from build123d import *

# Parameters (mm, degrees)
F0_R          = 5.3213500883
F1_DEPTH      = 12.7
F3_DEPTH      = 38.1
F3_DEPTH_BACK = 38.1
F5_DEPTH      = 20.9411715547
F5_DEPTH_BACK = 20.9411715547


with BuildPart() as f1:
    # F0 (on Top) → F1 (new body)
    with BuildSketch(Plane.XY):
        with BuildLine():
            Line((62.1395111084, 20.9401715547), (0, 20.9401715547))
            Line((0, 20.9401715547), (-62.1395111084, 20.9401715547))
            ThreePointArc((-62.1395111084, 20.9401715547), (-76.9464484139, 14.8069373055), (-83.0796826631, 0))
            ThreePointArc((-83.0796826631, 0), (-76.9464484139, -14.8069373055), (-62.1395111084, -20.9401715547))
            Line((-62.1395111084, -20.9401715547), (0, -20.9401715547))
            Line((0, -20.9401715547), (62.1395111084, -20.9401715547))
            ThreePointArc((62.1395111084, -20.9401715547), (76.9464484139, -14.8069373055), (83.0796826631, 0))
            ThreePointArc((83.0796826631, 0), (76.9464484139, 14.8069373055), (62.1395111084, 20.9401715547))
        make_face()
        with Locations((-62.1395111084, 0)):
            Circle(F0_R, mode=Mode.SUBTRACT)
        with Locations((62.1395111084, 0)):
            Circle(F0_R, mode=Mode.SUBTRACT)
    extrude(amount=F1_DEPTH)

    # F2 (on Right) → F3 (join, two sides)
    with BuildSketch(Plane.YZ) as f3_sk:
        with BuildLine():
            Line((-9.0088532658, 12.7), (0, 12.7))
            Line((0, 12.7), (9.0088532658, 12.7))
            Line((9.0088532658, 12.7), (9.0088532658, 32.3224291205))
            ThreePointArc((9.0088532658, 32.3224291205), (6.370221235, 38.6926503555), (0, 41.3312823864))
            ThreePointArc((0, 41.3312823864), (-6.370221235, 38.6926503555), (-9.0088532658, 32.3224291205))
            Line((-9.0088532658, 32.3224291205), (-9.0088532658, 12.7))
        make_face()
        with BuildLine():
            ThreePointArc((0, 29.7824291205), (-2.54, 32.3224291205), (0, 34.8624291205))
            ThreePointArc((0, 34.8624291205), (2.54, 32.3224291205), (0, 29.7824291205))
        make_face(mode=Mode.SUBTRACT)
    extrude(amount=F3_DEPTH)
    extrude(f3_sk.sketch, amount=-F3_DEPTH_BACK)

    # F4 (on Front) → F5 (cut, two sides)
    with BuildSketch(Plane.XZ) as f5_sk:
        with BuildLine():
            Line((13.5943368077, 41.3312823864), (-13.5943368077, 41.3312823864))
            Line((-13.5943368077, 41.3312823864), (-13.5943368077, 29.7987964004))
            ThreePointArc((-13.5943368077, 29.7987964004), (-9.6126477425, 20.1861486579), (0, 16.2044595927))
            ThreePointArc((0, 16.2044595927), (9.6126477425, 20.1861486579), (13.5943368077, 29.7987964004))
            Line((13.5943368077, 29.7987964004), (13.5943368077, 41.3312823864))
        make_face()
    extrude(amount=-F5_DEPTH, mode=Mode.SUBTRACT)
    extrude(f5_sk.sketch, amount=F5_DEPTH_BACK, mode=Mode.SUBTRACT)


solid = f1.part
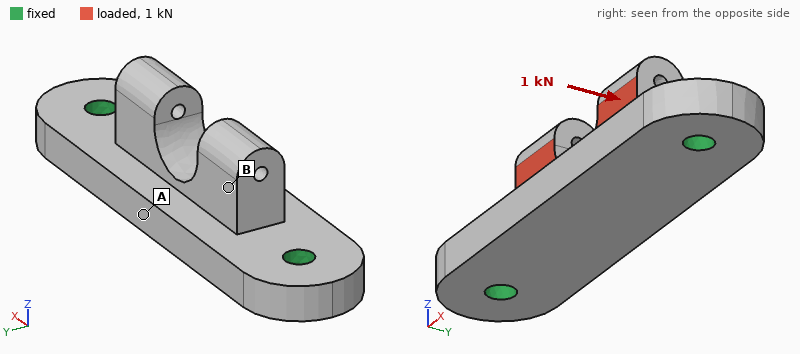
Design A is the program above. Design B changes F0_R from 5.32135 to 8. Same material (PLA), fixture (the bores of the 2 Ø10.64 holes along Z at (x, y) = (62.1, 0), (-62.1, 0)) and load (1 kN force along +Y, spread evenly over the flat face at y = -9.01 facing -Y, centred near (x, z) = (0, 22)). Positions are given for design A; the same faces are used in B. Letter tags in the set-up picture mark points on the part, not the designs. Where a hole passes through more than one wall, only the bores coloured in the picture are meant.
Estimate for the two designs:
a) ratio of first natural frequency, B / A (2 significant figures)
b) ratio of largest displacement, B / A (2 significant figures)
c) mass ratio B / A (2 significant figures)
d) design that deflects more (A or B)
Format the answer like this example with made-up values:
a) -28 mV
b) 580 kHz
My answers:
a) 1.1
b) 0.81
c) 0.97
d) A
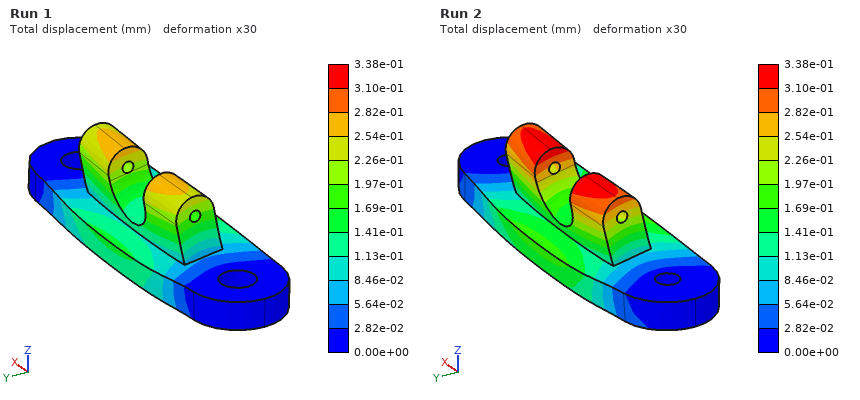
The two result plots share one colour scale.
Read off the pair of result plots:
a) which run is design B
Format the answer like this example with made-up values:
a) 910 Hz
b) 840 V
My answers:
a) Run 1
